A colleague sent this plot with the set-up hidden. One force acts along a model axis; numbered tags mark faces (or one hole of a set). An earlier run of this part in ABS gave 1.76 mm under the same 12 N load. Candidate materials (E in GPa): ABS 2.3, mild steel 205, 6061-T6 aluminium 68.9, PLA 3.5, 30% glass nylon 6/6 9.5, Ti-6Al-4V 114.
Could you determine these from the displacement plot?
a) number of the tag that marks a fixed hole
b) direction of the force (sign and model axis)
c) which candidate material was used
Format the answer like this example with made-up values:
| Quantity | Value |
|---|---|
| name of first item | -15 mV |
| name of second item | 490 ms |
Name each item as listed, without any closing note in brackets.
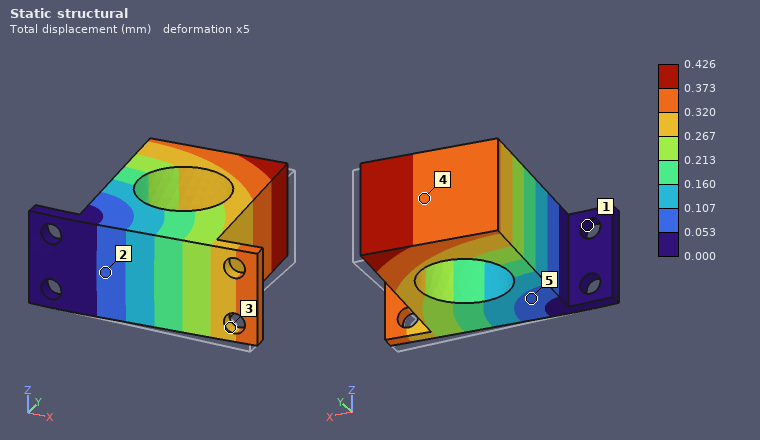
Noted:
| Quantity | Value |
|---|---|
| number of the tag that marks a fixed hole | 1 |
| direction of the force | +Y |
| which candidate material was used | 30% glass nylon 6/6 |
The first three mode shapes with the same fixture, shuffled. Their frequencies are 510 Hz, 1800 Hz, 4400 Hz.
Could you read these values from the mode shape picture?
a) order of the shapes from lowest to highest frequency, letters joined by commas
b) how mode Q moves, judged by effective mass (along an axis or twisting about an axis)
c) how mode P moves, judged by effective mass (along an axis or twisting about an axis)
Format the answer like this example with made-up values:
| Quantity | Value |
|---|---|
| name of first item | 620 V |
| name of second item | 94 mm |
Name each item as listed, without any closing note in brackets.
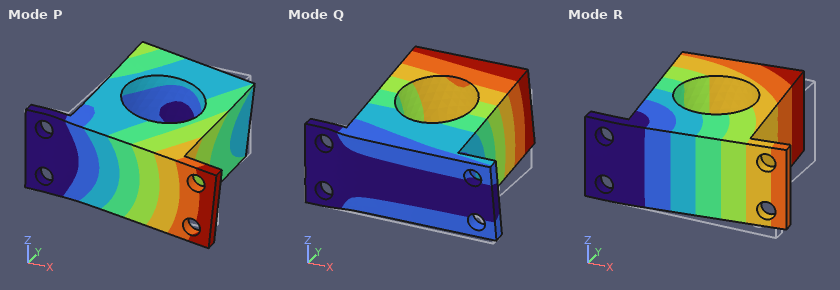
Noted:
| Quantity | Value |
|---|---|
| order of the shapes from lowest to highest frequency, letters joined by commas | R, Q, P |
| how mode Q moves, judged by effective mass | along Z |
| how mode P moves, judged by effective mass | along Z |
